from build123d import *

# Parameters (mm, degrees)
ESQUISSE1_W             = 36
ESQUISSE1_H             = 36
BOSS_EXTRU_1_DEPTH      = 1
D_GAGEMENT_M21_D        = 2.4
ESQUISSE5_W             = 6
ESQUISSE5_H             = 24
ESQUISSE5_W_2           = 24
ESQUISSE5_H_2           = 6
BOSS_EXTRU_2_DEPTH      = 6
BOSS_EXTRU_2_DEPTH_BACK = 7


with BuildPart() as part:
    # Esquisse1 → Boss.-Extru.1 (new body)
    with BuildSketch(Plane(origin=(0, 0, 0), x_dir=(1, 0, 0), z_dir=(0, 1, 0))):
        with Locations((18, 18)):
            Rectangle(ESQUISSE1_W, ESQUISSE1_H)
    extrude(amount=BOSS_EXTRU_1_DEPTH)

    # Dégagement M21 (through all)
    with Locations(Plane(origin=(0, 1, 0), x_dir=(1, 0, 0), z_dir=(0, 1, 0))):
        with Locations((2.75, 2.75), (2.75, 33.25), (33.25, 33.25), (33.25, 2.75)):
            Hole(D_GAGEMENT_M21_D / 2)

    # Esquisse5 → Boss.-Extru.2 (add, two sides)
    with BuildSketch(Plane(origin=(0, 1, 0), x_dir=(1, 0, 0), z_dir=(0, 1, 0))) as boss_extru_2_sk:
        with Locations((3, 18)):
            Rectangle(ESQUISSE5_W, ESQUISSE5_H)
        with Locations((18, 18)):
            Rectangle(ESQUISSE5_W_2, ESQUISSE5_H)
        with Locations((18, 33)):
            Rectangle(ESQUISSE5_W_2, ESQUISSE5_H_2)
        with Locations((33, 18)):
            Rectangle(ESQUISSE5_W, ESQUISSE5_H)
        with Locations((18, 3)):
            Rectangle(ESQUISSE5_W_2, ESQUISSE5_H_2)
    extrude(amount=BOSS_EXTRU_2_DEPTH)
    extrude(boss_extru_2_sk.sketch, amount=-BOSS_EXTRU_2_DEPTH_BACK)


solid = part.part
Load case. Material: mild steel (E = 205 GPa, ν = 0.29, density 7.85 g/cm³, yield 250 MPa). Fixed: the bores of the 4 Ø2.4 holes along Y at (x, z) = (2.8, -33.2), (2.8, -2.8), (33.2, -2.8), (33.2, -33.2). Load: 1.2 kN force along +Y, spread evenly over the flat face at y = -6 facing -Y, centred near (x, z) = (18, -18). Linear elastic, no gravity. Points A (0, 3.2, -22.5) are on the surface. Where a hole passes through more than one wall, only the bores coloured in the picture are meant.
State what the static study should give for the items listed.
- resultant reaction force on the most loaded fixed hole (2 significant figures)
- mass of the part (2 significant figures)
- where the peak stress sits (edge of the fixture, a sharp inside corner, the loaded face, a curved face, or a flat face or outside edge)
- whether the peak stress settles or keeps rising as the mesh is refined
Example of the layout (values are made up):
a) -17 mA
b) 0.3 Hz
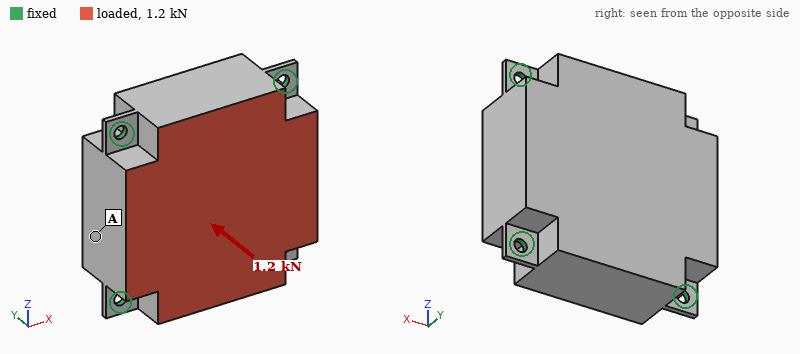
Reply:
a) 300 N
b) 120 g
c) edge of the fixture
d) keeps rising
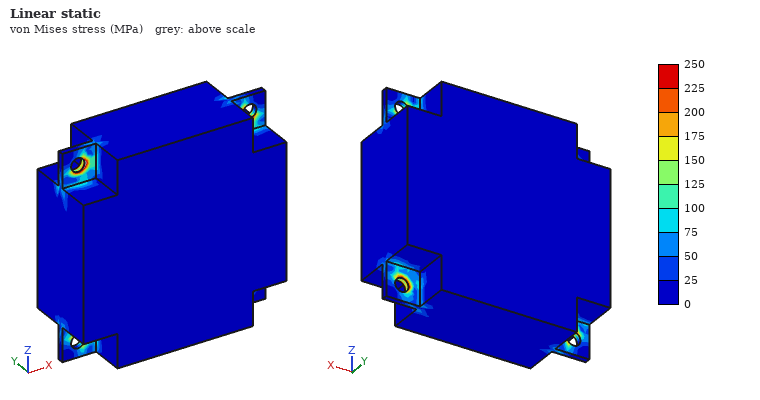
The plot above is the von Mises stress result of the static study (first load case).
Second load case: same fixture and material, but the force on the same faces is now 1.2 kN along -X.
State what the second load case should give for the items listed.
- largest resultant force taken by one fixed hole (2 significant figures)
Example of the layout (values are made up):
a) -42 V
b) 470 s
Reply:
a) 330 N
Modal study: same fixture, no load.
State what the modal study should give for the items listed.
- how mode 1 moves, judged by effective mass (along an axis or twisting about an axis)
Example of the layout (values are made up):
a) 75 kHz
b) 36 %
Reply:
a) along Y
